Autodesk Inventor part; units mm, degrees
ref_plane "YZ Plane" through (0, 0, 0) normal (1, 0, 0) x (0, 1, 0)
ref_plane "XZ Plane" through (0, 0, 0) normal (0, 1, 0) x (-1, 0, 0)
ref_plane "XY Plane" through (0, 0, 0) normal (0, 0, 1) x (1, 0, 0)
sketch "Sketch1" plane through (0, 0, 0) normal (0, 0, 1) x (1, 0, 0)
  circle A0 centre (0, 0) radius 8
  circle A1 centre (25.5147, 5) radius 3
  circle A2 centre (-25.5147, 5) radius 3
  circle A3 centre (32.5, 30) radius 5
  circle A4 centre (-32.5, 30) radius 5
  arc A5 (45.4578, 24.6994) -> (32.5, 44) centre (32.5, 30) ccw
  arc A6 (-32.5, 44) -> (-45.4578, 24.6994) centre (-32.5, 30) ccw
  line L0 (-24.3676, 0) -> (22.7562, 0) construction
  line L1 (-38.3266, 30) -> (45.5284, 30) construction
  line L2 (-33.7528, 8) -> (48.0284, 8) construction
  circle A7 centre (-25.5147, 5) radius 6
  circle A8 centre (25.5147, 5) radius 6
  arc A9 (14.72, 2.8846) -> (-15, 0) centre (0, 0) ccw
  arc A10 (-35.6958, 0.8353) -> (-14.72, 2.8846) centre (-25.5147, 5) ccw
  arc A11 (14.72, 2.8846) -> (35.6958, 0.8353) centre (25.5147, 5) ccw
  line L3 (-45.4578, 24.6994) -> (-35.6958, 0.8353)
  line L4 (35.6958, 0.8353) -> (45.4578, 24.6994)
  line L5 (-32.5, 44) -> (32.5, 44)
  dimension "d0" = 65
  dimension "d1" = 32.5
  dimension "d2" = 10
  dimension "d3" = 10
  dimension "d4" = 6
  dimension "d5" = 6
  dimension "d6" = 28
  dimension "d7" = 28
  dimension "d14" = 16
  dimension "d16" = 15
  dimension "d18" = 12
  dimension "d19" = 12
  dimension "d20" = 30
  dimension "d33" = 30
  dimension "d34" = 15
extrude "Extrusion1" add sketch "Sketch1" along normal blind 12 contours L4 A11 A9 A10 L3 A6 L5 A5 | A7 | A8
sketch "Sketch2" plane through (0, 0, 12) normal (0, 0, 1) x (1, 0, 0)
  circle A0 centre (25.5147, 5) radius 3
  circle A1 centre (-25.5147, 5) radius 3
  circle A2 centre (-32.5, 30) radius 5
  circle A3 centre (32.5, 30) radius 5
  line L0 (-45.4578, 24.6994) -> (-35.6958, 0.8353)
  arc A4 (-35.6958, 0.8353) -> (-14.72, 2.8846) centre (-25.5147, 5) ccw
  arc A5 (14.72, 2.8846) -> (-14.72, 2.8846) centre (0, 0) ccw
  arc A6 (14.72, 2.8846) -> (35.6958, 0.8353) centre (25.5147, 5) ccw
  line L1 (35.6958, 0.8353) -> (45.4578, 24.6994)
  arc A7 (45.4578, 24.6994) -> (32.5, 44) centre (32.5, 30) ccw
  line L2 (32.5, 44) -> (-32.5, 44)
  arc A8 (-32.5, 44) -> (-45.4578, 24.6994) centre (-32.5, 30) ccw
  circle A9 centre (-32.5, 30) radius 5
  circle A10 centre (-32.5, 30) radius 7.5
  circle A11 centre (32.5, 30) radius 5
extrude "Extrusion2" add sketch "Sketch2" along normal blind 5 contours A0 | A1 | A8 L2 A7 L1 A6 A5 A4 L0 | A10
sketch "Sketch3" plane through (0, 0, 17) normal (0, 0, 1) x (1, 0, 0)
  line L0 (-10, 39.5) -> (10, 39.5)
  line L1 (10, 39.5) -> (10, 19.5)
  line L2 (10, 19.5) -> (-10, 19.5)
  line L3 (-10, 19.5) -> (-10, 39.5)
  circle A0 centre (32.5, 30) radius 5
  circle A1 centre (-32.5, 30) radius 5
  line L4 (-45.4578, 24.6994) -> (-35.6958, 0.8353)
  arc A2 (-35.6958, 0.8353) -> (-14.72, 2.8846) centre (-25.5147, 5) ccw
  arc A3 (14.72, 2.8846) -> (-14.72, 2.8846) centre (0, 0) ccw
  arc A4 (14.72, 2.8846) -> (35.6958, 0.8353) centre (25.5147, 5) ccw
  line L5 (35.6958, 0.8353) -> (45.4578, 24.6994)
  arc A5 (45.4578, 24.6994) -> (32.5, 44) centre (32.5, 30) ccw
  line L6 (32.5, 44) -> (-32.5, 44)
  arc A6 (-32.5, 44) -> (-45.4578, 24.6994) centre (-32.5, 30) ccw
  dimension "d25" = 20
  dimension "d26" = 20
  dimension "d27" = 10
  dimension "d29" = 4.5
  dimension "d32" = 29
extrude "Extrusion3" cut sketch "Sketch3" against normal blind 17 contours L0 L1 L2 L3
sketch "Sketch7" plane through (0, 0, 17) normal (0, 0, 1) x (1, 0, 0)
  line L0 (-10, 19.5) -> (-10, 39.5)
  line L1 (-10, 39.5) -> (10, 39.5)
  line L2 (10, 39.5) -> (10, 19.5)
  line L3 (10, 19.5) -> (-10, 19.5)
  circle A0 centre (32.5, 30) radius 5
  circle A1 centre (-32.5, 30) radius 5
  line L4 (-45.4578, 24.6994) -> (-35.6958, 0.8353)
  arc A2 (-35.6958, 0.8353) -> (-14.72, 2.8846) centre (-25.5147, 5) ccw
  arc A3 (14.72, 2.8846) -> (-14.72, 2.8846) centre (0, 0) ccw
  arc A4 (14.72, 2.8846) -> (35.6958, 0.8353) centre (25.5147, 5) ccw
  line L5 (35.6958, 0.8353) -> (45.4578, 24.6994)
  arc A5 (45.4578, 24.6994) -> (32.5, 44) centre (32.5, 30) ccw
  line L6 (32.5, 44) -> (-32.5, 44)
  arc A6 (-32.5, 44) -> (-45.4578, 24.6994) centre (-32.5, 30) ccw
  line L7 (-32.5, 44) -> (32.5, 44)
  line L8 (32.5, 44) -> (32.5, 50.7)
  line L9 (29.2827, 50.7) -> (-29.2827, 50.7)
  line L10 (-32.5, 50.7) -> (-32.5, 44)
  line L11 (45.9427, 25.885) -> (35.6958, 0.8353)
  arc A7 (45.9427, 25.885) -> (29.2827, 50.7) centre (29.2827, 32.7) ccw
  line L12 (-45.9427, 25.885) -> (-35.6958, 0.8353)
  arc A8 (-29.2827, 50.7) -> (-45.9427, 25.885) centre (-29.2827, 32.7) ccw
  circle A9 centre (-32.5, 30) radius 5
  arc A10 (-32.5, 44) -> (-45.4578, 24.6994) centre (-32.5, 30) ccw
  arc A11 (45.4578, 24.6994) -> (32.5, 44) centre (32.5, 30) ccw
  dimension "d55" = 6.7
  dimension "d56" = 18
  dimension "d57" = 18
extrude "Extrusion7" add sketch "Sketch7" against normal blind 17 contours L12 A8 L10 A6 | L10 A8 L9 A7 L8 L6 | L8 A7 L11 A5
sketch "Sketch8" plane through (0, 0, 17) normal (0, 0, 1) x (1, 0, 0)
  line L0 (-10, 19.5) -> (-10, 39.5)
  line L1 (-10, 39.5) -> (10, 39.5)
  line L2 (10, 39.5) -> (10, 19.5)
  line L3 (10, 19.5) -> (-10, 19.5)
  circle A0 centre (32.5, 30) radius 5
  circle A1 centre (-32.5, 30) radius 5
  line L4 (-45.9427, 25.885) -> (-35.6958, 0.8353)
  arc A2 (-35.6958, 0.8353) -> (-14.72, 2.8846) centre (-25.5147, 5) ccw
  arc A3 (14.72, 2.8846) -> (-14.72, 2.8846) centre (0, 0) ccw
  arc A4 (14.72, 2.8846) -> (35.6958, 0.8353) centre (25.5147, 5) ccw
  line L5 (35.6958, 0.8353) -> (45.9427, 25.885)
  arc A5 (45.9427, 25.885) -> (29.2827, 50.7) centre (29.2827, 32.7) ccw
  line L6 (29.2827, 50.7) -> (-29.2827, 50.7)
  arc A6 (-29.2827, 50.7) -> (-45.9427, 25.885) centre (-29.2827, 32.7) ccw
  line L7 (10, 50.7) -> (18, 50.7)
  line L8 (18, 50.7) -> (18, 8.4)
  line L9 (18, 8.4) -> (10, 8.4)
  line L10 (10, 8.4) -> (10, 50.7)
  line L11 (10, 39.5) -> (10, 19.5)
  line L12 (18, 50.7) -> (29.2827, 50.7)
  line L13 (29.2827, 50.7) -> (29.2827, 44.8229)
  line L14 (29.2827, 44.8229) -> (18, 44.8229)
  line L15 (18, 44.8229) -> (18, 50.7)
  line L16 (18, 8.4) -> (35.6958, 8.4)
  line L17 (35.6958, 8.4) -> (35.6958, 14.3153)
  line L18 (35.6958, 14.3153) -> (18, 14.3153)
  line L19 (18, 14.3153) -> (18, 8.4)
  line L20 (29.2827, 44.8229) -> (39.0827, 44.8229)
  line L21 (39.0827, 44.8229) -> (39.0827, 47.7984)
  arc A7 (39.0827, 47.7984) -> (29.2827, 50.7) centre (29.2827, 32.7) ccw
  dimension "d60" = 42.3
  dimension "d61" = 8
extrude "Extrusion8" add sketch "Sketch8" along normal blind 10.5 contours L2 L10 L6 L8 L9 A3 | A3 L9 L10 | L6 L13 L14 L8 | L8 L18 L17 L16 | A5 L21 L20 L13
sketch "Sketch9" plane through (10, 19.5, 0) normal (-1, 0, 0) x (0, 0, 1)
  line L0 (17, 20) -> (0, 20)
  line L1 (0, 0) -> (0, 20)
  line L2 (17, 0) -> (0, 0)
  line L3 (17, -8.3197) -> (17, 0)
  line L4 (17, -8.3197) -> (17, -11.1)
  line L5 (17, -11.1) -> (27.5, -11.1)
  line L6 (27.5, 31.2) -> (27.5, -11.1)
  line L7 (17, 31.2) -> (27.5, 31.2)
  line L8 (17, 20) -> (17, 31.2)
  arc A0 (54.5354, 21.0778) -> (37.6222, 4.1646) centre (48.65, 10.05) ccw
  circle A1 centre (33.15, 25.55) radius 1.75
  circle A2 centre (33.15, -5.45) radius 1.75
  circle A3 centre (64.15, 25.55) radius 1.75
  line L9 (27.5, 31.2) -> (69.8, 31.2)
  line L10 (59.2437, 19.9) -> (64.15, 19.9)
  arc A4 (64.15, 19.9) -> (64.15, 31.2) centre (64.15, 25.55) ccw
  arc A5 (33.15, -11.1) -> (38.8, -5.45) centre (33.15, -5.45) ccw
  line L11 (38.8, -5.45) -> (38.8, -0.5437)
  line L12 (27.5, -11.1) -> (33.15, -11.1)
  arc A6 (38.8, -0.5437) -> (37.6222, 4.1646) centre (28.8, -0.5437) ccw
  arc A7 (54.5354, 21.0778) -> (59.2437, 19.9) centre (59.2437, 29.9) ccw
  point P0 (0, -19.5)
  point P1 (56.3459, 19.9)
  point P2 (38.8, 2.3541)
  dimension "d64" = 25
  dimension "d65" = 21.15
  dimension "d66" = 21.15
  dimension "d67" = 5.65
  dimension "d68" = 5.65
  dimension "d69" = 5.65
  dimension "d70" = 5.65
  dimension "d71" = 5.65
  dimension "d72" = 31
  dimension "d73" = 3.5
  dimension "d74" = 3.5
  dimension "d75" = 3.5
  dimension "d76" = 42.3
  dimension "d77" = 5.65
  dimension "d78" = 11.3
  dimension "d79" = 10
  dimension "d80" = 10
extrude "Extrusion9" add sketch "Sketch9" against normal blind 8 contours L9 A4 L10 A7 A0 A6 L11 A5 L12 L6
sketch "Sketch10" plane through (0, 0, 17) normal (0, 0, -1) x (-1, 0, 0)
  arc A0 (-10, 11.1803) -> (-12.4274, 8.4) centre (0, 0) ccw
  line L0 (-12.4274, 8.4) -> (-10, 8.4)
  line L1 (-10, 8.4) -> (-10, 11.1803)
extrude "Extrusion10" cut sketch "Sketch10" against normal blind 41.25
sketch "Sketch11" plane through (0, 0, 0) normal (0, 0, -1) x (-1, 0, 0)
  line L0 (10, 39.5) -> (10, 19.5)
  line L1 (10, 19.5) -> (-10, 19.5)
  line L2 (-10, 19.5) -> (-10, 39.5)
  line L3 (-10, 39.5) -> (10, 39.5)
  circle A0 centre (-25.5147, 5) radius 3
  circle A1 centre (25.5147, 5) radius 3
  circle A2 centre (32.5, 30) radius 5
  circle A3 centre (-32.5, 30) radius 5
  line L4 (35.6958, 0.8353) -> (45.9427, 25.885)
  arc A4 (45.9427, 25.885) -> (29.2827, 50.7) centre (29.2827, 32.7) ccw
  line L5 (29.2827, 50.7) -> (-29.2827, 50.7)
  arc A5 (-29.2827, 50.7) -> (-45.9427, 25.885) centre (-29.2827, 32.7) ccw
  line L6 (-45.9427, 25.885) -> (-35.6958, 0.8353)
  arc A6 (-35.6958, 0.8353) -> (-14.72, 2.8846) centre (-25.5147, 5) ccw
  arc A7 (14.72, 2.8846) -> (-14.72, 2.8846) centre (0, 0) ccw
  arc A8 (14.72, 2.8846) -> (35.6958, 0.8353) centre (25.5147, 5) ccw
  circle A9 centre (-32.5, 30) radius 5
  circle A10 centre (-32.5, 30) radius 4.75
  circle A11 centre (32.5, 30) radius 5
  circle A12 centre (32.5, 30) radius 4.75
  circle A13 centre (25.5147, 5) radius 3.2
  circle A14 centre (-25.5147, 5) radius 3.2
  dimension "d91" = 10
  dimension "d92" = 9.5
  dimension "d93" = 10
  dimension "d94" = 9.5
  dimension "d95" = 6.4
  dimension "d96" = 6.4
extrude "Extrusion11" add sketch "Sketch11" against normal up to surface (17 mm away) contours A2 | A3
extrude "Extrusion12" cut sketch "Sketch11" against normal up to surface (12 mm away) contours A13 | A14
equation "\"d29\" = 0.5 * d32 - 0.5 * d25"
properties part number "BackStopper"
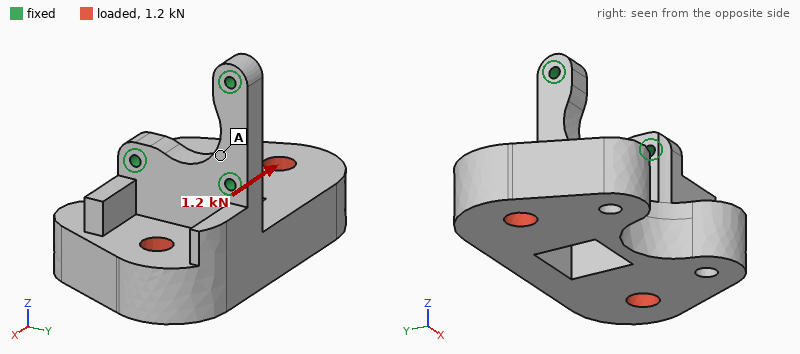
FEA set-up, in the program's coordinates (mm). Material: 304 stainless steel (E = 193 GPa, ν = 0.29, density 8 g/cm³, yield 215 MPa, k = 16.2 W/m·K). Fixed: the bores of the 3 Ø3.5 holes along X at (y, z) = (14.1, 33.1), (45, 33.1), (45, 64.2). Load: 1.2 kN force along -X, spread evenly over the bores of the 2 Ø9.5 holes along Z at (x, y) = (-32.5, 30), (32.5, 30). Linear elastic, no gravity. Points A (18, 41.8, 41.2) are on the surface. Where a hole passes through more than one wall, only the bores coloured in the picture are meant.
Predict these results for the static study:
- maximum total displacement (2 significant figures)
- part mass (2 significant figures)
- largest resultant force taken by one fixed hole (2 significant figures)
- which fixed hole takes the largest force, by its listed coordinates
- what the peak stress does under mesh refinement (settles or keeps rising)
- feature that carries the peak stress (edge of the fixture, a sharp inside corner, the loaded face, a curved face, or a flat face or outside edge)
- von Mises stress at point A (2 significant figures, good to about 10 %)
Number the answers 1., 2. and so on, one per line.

1. 75 µm
2. 570 g
3. 710 N
4. (45, 33.1)
5. keeps rising
6. edge of the fixture
7. 14 MPa
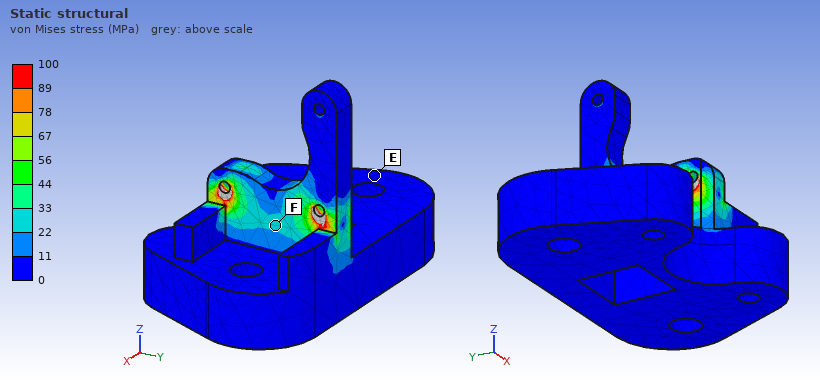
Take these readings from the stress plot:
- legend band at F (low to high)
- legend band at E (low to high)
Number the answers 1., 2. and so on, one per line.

1. 22 to 33 MPa
2. 0 to 11 MPa
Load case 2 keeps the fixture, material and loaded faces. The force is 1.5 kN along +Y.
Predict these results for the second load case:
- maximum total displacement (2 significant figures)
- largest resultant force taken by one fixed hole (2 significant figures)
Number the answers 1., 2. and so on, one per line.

1. 23 µm
2. 1.5 kN
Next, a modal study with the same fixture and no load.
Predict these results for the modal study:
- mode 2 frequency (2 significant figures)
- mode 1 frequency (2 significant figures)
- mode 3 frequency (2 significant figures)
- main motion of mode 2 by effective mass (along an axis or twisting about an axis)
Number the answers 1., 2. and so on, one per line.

1. 1900 Hz
2. 860 Hz
3. 3300 Hz
4. along Y
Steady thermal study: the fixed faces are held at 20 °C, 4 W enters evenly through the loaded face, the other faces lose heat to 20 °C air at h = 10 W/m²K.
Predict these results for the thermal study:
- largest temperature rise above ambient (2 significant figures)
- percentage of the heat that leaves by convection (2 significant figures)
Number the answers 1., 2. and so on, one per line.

1. 18 K
2. 44 %
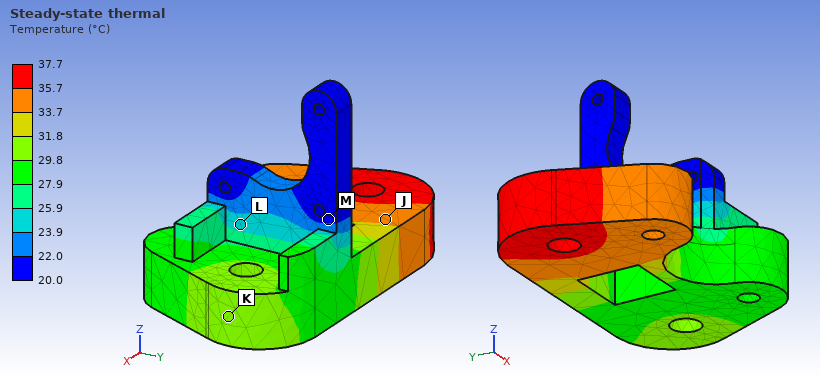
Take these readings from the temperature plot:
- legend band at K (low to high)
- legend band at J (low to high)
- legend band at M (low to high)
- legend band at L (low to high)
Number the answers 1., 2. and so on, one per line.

1. 29.8 to 31.8 °C
2. 33.7 to 35.7 °C
3. 20.0 to 22.0 °C
4. 23.9 to 25.9 °C
